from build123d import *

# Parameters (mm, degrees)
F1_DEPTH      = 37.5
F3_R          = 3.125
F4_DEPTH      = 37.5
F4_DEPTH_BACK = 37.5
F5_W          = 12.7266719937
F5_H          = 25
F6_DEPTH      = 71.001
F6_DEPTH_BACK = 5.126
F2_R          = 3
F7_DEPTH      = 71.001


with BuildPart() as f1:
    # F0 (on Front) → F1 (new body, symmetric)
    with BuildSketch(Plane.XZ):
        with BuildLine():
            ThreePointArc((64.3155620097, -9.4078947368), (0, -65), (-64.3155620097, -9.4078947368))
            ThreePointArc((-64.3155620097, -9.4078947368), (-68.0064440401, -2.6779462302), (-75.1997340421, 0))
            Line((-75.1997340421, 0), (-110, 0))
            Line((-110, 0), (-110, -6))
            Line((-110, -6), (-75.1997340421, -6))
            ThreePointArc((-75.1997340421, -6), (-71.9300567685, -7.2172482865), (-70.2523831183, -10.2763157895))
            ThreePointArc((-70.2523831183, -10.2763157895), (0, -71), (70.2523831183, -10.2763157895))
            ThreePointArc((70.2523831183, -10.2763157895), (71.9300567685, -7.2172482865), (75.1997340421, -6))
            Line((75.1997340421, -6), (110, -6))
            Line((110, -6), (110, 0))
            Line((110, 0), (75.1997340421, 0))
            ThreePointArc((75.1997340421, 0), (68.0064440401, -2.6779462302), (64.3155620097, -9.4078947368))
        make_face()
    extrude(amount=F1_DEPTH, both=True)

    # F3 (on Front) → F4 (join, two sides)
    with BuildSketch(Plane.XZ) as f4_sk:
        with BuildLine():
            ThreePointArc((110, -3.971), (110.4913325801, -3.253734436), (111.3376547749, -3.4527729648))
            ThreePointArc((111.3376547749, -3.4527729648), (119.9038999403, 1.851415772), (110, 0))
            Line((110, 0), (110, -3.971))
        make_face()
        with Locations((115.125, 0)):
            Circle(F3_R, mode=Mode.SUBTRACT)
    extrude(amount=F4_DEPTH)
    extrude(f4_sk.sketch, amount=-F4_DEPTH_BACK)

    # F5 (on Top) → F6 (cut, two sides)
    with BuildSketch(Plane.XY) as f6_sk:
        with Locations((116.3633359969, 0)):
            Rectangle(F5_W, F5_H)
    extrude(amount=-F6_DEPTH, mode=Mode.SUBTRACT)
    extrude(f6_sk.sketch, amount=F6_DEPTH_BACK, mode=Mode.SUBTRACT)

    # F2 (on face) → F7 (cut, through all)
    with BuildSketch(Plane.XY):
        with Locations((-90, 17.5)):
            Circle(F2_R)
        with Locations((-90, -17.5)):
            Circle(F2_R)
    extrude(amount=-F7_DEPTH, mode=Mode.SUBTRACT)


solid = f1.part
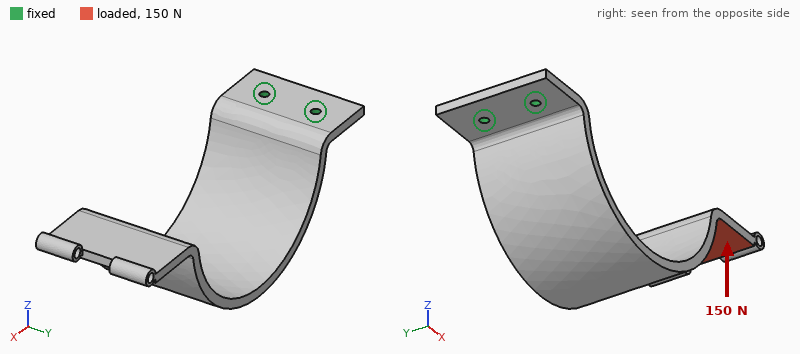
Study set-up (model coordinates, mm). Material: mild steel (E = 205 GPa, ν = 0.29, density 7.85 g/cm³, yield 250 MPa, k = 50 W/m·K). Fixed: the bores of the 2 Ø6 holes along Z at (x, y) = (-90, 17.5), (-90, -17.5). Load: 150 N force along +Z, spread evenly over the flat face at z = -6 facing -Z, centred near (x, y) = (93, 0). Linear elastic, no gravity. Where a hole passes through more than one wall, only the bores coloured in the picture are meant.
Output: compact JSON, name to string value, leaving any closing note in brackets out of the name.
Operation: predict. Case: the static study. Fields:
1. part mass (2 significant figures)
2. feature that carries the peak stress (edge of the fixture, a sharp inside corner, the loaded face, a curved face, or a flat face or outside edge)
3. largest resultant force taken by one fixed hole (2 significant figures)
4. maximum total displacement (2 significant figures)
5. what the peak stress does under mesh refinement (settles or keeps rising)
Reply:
{"part mass": "1.0 kg", "feature that carries the peak stress": "edge of the fixture", "largest resultant force taken by one fixed hole": "78 N", "maximum total displacement": "1.9 mm", "what the peak stress does under mesh refinement": "keeps rising"}
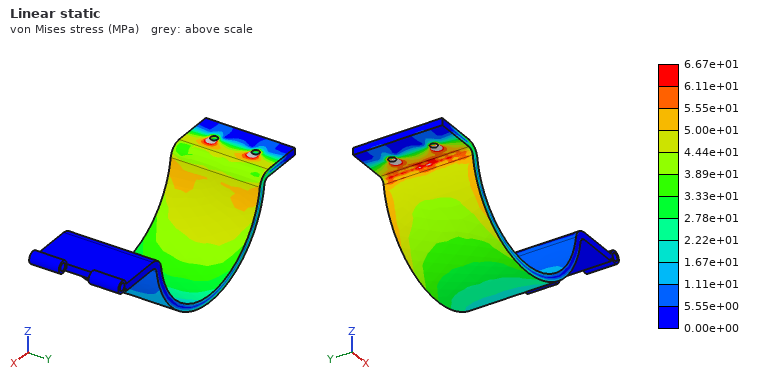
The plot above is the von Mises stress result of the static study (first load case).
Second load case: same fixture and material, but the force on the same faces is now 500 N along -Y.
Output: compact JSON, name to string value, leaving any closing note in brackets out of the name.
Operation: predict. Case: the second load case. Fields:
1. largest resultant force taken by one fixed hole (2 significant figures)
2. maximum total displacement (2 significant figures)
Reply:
{"largest resultant force taken by one fixed hole": "2.4 kN", "maximum total displacement": "2.2 mm"}
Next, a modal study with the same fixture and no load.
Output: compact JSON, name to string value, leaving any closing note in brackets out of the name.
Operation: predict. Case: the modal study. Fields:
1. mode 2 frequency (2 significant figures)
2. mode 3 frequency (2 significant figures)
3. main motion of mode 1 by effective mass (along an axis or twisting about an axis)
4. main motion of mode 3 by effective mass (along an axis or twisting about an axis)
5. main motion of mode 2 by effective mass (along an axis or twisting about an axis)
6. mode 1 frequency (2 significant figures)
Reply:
{"mode 2 frequency": "150 Hz", "mode 3 frequency": "270 Hz", "main motion of mode 1 by effective mass": "along Z", "main motion of mode 3 by effective mass": "along X", "main motion of mode 2 by effective mass": "along Y", "mode 1 frequency": "86 Hz"}
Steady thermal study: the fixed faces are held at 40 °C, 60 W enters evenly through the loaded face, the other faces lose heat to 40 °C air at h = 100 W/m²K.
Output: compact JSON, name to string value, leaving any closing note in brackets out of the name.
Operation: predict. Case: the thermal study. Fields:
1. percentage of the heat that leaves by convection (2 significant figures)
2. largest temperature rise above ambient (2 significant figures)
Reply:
{"percentage of the heat that leaves by convection": "100 %", "largest temperature rise above ambient": "65 K"}
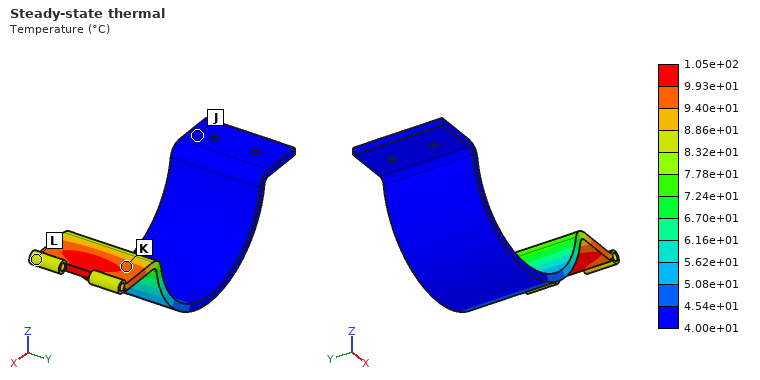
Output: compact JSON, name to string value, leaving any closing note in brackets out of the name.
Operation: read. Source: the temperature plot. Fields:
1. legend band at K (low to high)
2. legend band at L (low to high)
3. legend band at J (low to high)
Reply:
{"legend band at K": "9.40e+01 to 9.93e+01 °C", "legend band at L": "8.32e+01 to 8.86e+01 °C", "legend band at J": "4.00e+01 to 4.54e+01 °C"}
